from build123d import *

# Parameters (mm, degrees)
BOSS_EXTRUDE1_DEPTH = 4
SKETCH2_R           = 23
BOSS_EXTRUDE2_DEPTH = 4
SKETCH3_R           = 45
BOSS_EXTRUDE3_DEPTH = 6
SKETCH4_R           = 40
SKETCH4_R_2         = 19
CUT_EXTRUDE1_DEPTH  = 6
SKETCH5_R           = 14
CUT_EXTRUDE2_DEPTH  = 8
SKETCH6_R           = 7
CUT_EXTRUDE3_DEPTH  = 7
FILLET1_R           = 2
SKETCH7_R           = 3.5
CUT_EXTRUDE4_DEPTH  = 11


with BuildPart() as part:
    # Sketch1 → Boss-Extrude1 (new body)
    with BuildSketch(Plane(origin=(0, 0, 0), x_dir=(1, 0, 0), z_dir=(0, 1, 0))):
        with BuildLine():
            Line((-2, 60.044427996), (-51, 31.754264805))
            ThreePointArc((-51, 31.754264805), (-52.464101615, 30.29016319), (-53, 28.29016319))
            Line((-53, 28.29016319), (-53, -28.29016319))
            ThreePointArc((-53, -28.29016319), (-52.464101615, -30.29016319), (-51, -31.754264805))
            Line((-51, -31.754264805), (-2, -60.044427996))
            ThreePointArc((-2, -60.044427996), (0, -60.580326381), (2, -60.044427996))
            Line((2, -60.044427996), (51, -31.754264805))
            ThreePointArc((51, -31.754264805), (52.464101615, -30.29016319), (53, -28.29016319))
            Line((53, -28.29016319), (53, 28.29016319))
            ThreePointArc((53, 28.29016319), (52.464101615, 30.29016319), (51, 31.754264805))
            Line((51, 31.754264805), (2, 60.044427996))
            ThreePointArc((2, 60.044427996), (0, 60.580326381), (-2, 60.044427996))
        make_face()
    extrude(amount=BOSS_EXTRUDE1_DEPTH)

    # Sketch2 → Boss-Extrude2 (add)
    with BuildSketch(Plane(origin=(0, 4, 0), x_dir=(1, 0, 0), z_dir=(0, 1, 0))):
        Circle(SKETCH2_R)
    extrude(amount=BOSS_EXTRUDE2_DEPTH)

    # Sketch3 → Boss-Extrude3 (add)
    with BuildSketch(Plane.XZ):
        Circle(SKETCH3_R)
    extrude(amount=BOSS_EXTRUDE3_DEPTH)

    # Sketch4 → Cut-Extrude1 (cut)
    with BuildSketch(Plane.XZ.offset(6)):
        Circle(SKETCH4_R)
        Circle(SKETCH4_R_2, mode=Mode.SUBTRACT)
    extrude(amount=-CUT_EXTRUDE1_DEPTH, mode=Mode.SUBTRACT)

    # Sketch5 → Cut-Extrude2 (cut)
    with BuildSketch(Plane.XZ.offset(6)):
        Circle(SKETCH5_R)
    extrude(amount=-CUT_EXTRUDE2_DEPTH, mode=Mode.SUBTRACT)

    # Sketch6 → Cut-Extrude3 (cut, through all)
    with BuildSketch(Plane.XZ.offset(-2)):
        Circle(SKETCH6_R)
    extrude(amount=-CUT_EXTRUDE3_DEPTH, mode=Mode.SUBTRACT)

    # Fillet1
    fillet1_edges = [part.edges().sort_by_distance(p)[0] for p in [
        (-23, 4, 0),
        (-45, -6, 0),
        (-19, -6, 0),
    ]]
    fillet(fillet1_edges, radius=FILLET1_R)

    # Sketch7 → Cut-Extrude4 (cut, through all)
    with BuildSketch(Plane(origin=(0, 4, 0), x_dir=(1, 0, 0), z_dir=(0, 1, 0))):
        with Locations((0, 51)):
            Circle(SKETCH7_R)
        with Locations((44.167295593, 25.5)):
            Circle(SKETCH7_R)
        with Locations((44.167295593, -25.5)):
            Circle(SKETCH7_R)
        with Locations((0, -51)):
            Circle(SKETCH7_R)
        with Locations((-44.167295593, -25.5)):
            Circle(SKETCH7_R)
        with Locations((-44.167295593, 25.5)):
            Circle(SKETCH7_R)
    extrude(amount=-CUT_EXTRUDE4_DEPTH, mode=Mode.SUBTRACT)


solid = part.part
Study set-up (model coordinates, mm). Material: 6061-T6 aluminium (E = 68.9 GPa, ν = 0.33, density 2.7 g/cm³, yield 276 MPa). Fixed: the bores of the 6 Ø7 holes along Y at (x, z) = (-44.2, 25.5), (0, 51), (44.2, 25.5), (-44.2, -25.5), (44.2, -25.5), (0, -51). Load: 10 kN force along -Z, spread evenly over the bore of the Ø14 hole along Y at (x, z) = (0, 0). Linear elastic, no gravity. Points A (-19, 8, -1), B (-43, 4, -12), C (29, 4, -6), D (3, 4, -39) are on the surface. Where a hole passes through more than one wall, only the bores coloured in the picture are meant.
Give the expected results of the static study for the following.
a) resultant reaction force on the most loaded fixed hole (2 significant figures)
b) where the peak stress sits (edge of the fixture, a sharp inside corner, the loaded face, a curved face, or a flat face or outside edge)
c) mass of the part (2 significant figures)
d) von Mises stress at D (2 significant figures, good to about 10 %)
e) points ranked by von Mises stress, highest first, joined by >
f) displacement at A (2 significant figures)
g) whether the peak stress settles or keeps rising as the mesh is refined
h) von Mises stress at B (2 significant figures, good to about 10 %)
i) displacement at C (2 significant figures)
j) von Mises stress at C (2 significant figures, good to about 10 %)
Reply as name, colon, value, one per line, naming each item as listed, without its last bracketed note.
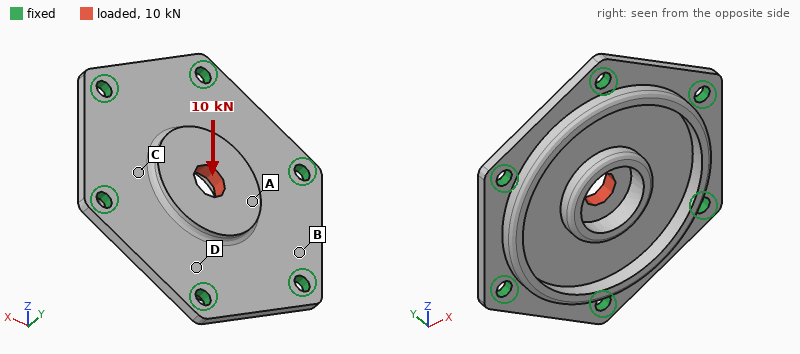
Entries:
resultant reaction force on the most loaded fixed hole: 2.5 kN
where the peak stress sits: edge of the fixture
mass of the part: 140 g
von Mises stress at D: 29 MPa
points ranked by von Mises stress, highest first, joined by >: D > C > B > A
displacement at A: 14 µm
whether the peak stress settles or keeps rising as the mesh is refined: keeps rising
von Mises stress at B: 12 MPa
displacement at C: 7.4 µm
von Mises stress at C: 21 MPa
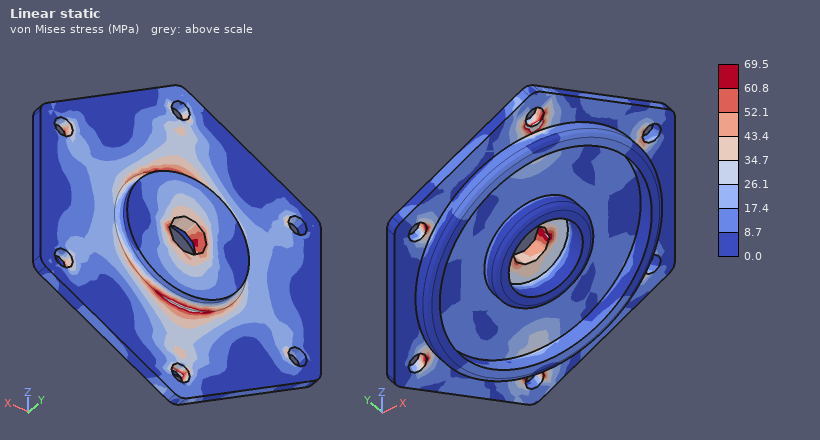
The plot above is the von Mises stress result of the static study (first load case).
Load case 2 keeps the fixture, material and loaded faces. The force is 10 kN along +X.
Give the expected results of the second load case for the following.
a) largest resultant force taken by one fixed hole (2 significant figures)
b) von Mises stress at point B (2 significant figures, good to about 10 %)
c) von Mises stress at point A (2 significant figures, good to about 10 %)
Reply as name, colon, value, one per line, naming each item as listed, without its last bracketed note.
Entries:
largest resultant force taken by one fixed hole: 2.2 kN
von Mises stress at point B: 12 MPa
von Mises stress at point A: 19 MPa
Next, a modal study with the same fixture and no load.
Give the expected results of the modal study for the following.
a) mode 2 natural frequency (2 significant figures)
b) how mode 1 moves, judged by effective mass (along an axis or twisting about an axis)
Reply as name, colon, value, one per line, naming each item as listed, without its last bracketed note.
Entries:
mode 2 natural frequency: 7600 Hz
how mode 1 moves, judged by effective mass: along Y
